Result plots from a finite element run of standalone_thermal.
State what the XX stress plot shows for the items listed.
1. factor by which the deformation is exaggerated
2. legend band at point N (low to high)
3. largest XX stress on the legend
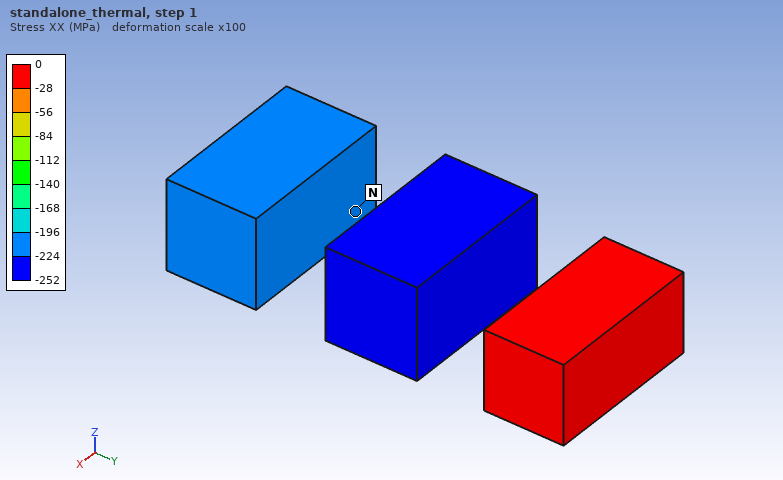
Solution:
100
-224 to -196 MPa
0 MPa
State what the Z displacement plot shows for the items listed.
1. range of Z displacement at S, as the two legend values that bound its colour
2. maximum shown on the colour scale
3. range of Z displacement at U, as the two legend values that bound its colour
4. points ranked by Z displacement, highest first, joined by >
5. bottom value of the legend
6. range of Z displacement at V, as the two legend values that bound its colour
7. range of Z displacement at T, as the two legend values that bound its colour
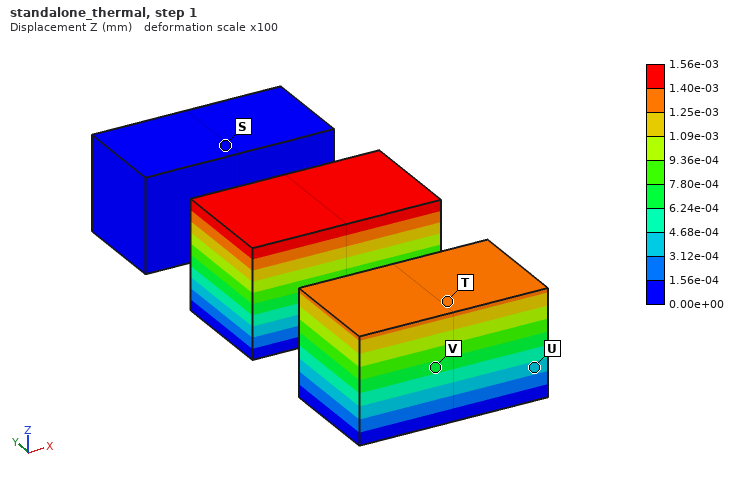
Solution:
0.00e+00 to 1.56e-04 mm
1.56e-03 mm
3.12e-04 to 4.68e-04 mm
T > V > U > S
0.00e+00 mm
6.24e-04 to 7.80e-04 mm
1.25e-03 to 1.40e-03 mm
